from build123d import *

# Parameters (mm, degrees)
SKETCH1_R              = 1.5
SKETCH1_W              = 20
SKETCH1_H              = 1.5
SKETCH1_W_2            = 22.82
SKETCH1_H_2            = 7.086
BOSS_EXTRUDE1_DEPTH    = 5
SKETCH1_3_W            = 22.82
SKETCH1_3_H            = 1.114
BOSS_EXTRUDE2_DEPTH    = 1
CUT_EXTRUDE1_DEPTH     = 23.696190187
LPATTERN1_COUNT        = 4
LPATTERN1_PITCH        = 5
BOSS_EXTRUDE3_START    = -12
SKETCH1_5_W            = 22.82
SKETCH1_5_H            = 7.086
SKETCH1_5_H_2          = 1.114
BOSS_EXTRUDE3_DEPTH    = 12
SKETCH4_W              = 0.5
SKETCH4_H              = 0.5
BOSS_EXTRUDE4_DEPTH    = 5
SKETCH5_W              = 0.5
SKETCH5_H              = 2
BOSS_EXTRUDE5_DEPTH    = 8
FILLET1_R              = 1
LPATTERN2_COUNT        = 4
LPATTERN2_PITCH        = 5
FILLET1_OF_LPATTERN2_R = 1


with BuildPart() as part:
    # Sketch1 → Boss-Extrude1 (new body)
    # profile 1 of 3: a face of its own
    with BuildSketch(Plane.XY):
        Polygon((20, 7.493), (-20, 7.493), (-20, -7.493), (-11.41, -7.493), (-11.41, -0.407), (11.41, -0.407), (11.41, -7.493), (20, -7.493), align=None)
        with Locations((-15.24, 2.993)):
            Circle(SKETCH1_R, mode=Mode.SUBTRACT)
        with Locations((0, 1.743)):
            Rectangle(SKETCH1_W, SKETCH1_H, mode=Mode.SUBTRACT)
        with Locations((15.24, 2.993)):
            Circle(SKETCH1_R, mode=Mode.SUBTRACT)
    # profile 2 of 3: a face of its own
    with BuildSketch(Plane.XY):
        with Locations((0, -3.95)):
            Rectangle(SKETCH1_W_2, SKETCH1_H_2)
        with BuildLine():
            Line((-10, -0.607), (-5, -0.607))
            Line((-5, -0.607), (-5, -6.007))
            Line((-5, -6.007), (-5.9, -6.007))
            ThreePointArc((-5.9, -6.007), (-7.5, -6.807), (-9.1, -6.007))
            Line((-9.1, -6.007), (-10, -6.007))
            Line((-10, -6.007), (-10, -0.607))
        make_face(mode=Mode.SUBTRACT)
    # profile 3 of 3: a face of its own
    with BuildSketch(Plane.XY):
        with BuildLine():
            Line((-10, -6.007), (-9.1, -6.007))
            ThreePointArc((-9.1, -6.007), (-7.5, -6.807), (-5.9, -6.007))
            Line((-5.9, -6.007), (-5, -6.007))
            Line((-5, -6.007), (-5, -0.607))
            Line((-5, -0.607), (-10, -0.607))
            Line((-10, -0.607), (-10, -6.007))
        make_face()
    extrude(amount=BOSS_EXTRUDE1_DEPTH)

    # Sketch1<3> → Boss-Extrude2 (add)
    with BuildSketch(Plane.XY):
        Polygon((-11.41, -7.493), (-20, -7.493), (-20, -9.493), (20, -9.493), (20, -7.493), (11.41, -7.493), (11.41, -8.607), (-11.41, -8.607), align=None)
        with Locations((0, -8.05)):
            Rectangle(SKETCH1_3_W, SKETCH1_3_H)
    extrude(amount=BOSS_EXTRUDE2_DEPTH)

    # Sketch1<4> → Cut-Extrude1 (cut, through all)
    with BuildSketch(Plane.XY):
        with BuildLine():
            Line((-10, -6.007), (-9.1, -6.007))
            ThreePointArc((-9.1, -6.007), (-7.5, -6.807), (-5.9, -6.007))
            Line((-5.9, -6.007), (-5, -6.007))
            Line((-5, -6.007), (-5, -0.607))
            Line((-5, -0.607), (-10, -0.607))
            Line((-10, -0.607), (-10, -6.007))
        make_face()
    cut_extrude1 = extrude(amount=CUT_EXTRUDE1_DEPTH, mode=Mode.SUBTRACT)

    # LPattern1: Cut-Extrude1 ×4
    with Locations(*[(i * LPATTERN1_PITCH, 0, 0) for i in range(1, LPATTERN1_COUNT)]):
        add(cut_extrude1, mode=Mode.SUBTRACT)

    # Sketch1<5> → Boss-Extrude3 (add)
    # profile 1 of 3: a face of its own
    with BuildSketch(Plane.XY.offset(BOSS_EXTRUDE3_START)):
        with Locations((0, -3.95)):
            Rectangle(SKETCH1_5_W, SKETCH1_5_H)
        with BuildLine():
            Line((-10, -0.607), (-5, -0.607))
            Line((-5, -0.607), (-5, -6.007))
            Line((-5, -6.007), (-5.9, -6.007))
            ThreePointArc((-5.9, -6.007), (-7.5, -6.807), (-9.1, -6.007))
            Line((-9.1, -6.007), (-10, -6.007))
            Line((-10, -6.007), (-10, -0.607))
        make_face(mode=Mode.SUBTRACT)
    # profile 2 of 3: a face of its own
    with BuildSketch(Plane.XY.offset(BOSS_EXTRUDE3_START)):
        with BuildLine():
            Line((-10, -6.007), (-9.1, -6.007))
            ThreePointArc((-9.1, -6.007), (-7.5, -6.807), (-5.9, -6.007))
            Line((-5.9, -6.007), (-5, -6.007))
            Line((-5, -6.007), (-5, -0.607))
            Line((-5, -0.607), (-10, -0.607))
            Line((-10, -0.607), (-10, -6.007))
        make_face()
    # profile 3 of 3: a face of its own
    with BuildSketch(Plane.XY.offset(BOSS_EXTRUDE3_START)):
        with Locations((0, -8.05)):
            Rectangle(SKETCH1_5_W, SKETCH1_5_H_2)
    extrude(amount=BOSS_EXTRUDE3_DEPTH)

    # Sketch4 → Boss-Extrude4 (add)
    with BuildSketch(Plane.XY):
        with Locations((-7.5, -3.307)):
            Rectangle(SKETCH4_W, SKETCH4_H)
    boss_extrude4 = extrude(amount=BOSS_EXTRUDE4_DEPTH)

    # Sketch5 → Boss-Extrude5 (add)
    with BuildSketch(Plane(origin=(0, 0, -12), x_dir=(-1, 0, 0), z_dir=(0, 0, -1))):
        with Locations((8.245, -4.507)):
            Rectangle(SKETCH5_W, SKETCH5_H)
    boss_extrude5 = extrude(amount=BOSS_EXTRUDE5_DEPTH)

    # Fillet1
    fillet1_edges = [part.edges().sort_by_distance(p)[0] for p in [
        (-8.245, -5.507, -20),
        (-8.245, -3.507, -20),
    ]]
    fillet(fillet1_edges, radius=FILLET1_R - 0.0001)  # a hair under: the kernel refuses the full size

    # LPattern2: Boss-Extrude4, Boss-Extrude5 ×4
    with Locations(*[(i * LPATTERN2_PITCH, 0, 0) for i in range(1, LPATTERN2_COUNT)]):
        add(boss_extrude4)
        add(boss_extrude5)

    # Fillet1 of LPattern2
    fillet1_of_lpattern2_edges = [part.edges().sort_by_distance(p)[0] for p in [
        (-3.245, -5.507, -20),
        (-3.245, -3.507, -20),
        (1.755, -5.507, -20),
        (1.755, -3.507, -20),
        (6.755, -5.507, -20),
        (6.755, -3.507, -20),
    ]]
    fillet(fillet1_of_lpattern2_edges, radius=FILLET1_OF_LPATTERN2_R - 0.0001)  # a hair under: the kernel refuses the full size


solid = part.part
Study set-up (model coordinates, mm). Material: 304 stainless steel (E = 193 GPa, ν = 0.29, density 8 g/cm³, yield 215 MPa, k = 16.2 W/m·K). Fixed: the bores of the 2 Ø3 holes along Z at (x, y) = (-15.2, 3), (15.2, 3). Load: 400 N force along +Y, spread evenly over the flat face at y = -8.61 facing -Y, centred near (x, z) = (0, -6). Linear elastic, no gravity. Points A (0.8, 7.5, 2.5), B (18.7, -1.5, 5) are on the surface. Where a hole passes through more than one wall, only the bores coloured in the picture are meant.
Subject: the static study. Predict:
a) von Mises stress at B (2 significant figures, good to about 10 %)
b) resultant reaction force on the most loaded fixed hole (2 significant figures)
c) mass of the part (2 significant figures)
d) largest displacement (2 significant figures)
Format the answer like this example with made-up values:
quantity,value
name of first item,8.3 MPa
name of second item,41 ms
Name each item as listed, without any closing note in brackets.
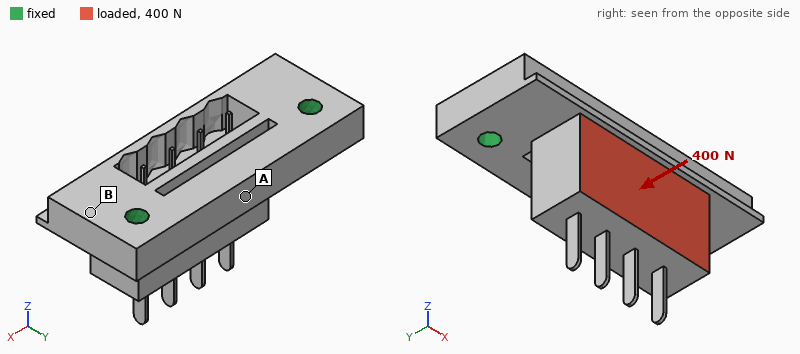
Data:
quantity,value
von Mises stress at B,23 MPa
resultant reaction force on the most loaded fixed hole,210 N
mass of the part,36 g
largest displacement,21 µm
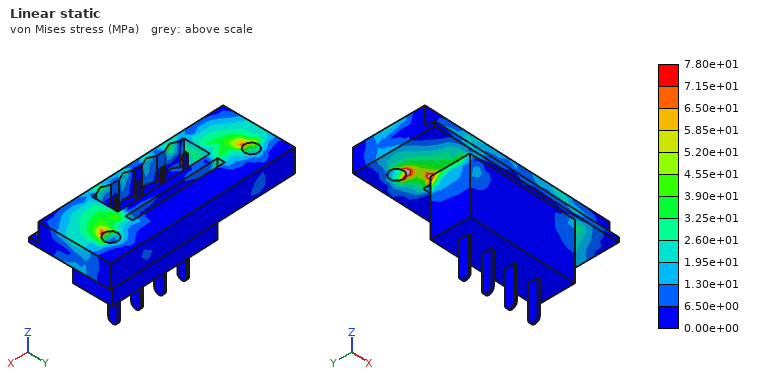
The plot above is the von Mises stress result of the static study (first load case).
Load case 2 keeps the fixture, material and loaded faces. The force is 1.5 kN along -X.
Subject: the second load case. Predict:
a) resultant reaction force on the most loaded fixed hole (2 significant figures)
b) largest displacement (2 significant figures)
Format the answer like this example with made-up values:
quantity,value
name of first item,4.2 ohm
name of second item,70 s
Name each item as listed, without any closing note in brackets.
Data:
quantity,value
resultant reaction force on the most loaded fixed hole,990 N
largest displacement,7.2 µm
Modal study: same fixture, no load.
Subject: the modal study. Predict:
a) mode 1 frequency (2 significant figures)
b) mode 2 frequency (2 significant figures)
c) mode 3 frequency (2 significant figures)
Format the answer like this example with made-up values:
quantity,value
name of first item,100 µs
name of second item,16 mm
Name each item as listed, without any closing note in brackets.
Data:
quantity,value
mode 1 frequency,6400 Hz
mode 2 frequency,6400 Hz
mode 3 frequency,6400 Hz
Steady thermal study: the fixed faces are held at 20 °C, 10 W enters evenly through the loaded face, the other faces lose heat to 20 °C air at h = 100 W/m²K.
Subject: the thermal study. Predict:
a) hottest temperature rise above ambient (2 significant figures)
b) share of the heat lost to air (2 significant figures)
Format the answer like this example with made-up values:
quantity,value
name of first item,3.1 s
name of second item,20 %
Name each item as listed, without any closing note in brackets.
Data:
quantity,value
hottest temperature rise above ambient,56 K
share of the heat lost to air,64 %
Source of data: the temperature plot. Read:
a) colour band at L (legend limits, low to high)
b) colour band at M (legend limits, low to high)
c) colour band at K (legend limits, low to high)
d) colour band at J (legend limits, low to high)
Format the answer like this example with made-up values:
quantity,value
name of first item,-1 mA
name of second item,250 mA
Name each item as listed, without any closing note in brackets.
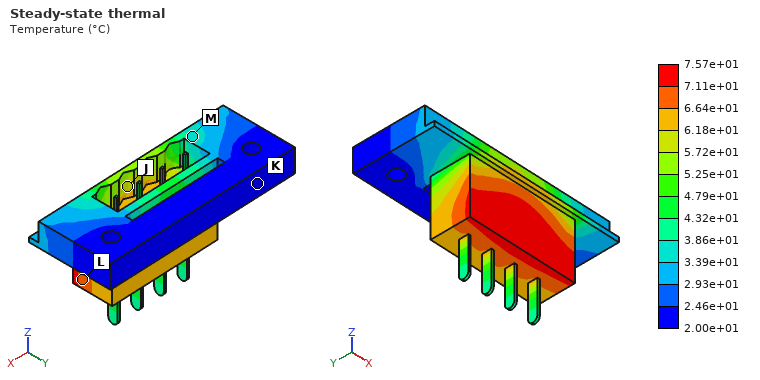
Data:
quantity,value
colour band at L,6.64e+01 to 7.11e+01 °C
colour band at M,3.39e+01 to 3.86e+01 °C
colour band at K,2.00e+01 to 2.46e+01 °C
colour band at J,5.72e+01 to 6.18e+01 °C
